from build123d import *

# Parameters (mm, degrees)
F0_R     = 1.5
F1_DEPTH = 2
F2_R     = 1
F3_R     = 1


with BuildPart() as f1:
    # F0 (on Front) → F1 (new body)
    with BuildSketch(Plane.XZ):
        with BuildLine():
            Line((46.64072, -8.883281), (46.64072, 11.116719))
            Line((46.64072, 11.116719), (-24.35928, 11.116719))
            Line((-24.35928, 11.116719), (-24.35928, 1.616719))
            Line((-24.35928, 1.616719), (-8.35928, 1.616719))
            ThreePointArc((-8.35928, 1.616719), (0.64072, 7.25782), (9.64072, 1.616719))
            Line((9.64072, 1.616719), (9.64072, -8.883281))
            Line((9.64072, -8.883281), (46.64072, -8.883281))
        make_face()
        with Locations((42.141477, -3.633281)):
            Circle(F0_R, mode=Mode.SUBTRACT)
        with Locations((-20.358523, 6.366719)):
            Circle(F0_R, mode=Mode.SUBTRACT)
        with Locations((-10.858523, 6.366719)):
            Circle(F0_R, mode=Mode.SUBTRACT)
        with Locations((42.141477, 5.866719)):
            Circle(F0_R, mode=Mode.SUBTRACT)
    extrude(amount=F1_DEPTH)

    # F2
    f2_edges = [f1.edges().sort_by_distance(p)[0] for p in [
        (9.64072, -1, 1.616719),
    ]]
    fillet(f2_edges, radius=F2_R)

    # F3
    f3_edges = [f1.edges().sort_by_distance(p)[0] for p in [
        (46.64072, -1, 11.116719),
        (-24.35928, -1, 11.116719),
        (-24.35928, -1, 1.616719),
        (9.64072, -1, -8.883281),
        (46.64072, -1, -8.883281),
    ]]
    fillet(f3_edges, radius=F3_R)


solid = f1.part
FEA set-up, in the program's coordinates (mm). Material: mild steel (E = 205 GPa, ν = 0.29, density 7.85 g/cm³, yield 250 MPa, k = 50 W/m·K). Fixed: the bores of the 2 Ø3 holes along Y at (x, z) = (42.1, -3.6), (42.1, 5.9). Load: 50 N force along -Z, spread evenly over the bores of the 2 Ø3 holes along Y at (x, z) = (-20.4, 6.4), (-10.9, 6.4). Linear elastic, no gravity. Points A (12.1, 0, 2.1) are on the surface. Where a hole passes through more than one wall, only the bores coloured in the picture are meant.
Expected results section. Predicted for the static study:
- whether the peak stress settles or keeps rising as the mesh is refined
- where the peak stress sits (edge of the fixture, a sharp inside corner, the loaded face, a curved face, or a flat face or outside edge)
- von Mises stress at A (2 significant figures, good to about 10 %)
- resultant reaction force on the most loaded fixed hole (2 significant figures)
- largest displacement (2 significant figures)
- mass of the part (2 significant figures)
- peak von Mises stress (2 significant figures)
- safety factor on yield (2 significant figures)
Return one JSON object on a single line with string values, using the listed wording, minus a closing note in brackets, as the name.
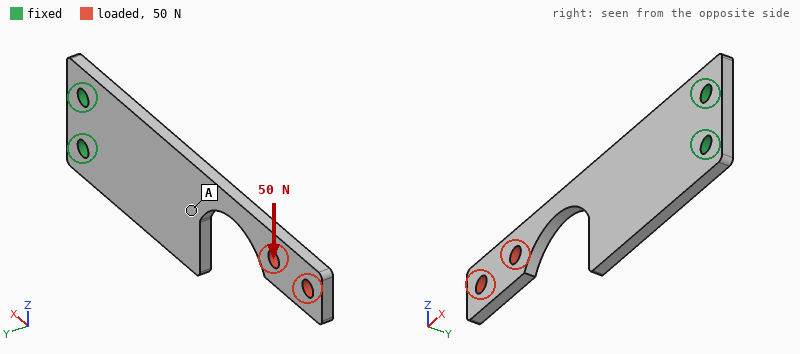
{"whether the peak stress settles or keeps rising as the mesh is refined": "settles", "where the peak stress sits": "a curved face", "von Mises stress at A": "20 MPa", "resultant reaction force on the most loaded fixed hole": "250 N", "largest displacement": "0.14 mm", "mass of the part": "15 g", "peak von Mises stress": "190 MPa", "safety factor on yield": "1.3"}
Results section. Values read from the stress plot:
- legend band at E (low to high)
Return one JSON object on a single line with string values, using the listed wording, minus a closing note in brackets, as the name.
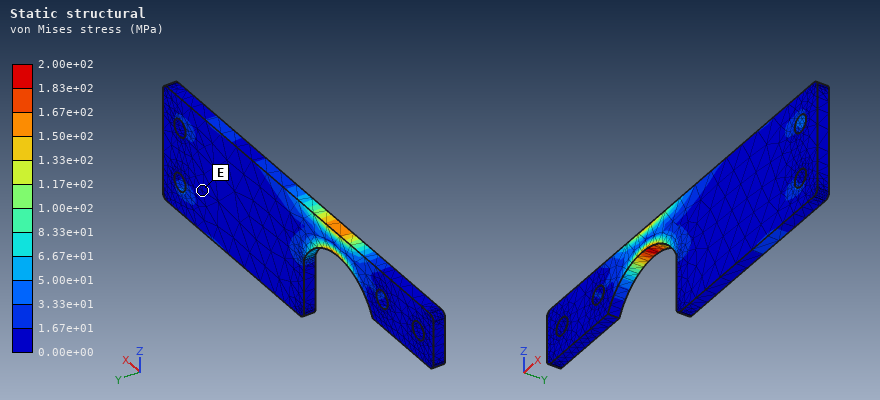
{"legend band at E": "0.00e+00 to 1.67e+01 MPa"}
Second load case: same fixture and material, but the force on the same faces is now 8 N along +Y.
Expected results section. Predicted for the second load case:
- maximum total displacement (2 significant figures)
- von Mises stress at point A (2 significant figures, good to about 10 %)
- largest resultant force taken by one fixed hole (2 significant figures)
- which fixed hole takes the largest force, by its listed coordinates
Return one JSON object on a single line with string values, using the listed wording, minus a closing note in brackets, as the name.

{"maximum total displacement": "0.32 mm", "von Mises stress at point A": "29 MPa", "largest resultant force taken by one fixed hole": "7.2 N", "which fixed hole takes the largest force, by its listed coordinates": "(42.1, 5.9)"}
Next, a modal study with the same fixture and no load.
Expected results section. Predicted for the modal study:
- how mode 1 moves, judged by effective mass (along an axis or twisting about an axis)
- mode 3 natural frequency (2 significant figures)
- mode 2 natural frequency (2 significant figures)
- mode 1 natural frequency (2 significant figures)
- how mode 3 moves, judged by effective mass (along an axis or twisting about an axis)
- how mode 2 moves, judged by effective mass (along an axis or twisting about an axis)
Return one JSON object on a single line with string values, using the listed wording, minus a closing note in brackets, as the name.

{"how mode 1 moves, judged by effective mass": "along Y", "mode 3 natural frequency": "2200 Hz", "mode 2 natural frequency": "2100 Hz", "mode 1 natural frequency": "530 Hz", "how mode 3 moves, judged by effective mass": "along Z", "how mode 2 moves, judged by effective mass": "along Y"}
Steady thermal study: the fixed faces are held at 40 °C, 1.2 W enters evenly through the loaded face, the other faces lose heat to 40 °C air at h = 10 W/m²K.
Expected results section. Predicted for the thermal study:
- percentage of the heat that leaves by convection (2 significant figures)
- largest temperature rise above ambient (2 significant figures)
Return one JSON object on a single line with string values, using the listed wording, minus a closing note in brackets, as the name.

{"percentage of the heat that leaves by convection": "33 %", "largest temperature rise above ambient": "62 K"}
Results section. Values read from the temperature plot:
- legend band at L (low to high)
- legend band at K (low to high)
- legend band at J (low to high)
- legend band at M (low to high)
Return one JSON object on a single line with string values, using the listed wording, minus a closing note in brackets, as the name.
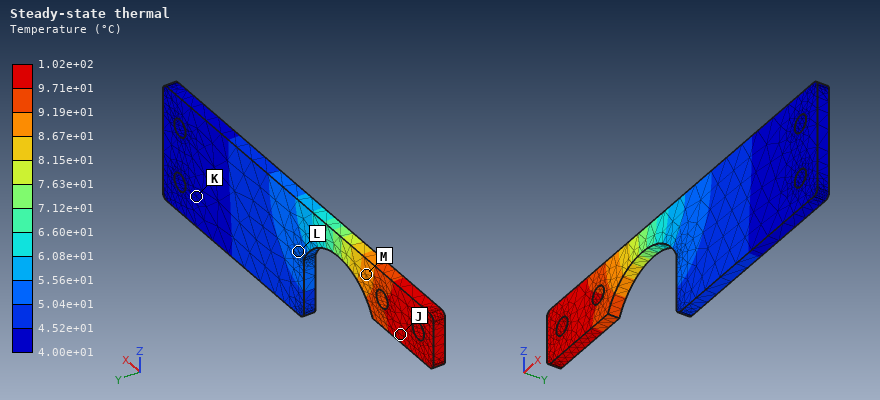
{"legend band at L": "5.04e+01 to 5.56e+01 °C", "legend band at K": "4.00e+01 to 4.52e+01 °C", "legend band at J": "9.71e+01 to 1.02e+02 °C", "legend band at M": "8.67e+01 to 9.19e+01 °C"}
